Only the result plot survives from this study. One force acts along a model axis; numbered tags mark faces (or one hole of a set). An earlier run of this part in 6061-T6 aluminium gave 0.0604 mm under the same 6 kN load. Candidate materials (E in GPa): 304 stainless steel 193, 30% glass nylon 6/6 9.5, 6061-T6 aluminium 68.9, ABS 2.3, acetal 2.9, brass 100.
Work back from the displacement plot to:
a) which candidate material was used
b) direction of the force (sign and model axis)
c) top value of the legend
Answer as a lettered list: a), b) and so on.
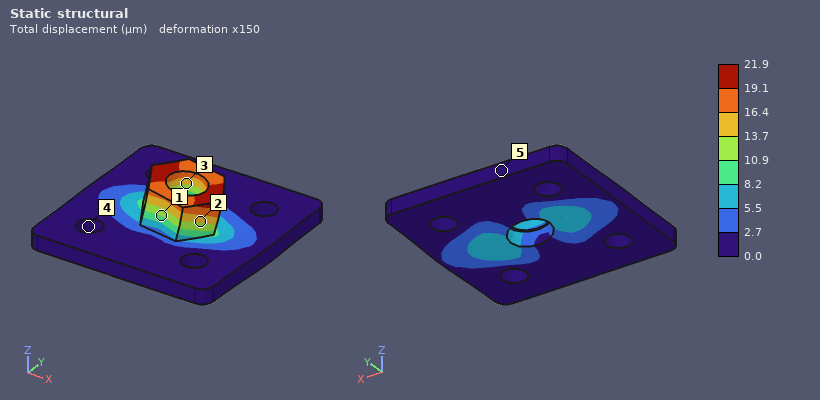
a) 304 stainless steel
b) +X
c) 21.9 µm
